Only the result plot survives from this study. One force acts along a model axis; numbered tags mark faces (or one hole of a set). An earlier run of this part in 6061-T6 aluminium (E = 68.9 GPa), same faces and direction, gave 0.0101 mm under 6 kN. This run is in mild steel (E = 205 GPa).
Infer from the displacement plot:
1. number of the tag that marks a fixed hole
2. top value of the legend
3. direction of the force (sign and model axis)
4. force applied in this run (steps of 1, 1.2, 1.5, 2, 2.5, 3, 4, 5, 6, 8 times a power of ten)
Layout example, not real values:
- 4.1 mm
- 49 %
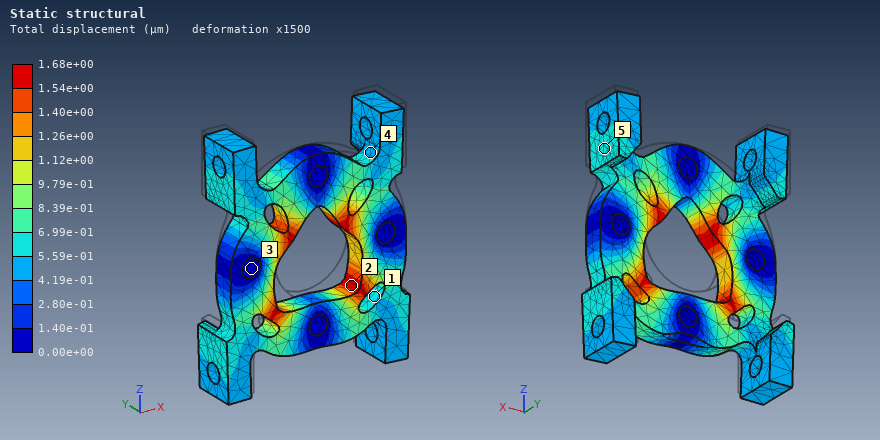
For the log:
- 3
- 1.68e+00 µm
- -Z
- 3 kN
